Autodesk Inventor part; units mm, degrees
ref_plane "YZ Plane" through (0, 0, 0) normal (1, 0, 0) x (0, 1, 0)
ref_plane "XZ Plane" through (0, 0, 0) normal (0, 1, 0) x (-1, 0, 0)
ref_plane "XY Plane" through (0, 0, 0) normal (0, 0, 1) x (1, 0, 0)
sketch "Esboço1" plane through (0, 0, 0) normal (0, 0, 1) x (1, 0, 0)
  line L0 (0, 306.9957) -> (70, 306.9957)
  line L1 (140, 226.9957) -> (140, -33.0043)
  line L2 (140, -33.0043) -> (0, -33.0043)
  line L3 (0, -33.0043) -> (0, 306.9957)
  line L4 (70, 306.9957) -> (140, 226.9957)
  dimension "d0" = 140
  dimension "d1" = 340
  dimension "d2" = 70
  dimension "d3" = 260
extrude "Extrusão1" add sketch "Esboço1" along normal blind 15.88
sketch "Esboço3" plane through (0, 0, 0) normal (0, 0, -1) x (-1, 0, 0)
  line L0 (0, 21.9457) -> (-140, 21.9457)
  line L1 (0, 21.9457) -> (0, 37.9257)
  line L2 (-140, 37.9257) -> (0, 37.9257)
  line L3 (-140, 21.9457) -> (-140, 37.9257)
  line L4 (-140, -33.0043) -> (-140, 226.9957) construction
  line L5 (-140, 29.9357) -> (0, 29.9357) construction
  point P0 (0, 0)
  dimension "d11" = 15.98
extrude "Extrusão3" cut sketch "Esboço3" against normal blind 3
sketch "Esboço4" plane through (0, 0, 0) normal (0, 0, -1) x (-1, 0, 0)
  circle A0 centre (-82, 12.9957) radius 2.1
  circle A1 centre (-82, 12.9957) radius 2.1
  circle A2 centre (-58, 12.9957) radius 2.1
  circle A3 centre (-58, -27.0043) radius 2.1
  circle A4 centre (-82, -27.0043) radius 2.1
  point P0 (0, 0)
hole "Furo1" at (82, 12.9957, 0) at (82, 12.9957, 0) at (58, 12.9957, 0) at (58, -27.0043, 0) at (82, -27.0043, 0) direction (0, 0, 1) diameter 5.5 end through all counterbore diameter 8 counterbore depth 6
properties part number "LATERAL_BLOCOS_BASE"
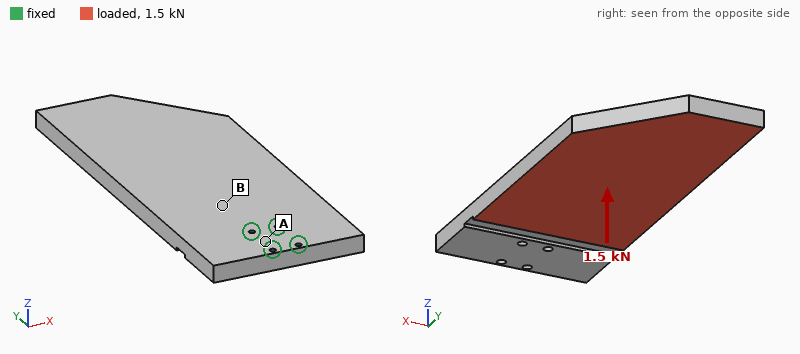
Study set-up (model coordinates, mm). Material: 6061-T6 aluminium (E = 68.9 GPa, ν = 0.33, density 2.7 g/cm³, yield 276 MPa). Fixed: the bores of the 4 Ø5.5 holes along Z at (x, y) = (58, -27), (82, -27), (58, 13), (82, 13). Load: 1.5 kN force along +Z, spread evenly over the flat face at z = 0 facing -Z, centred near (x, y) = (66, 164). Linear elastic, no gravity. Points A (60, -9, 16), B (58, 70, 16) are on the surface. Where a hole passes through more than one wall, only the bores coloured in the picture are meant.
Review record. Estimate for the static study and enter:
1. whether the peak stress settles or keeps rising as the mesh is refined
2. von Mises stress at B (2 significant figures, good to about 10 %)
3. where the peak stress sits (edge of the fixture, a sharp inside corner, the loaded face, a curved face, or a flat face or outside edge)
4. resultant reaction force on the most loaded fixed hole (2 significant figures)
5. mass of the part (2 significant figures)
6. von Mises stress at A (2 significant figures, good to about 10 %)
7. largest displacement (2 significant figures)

keeps rising
22 MPa
edge of the fixture
3.3 kN
1.9 kg
9.8 MPa
2.1 mm
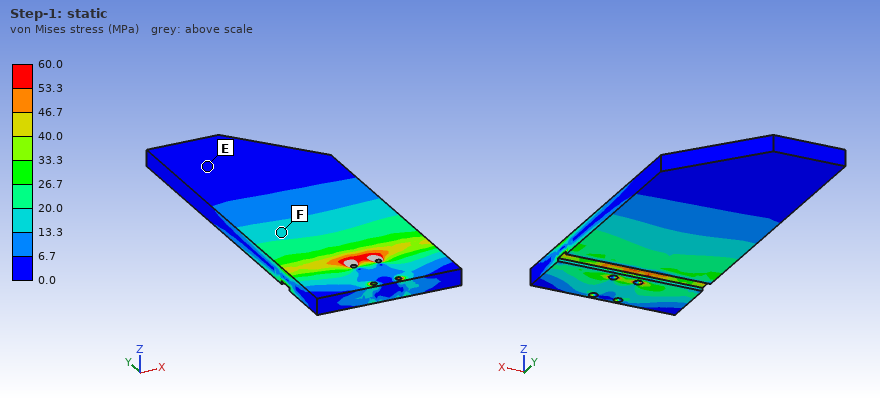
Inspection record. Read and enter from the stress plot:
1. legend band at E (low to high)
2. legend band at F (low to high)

0.0 to 6.7 MPa
13.3 to 20.0 MPa
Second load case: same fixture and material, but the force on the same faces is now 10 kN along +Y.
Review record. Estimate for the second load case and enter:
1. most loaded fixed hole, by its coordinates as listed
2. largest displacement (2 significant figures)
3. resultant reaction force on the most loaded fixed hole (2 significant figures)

(58, 13)
1.0 mm
3.7 kN
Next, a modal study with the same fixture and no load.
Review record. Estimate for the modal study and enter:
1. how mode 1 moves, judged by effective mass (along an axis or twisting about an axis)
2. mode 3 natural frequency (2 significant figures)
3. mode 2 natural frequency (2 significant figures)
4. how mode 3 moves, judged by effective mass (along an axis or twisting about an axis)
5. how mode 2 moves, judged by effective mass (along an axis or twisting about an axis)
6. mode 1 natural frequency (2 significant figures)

along Z
720 Hz
600 Hz
along X
twisting about Y
140 Hz
